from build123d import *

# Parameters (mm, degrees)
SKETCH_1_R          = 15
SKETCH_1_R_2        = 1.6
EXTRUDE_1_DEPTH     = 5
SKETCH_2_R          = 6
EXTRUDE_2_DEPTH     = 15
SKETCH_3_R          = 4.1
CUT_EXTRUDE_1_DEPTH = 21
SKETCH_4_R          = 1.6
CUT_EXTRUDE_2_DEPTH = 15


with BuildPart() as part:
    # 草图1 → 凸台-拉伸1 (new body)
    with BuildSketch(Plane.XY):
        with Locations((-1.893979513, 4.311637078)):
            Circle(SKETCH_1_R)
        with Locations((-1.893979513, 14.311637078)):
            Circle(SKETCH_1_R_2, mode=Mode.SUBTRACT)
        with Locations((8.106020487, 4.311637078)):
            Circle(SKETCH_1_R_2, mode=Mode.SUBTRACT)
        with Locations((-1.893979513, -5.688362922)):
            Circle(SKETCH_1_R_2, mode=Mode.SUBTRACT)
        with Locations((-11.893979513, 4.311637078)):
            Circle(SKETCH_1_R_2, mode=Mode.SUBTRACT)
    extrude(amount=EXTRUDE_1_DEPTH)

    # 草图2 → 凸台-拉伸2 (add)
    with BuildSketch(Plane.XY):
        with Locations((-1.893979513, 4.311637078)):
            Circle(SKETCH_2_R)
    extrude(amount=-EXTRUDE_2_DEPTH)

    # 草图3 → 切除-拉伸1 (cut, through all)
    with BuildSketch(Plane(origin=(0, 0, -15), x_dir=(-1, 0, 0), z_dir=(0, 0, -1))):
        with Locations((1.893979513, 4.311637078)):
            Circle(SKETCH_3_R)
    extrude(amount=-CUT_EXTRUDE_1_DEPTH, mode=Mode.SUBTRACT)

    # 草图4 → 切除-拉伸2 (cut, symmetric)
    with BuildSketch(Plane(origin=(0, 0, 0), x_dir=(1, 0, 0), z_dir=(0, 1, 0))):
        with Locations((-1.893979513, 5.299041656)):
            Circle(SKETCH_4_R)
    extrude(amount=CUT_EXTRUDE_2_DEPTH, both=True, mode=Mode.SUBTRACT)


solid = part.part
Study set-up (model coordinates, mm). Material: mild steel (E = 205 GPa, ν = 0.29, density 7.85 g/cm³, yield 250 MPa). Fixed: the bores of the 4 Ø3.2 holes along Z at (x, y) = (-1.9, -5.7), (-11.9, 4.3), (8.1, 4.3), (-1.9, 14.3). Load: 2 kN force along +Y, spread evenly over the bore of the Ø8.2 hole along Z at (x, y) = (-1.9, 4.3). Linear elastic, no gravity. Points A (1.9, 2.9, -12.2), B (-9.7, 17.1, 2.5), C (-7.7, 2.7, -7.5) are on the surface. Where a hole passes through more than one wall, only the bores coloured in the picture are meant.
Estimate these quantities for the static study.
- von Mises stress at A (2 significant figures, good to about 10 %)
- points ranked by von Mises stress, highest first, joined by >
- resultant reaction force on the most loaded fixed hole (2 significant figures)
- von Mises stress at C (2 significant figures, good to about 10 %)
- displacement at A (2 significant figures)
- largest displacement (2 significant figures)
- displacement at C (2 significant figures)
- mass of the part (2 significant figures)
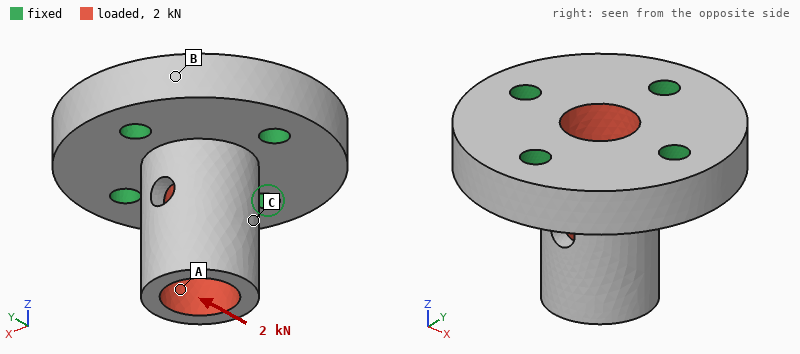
22 MPa
C > A > B
1.0 kN
43 MPa
12 µm
15 µm
7.5 µm
31 g
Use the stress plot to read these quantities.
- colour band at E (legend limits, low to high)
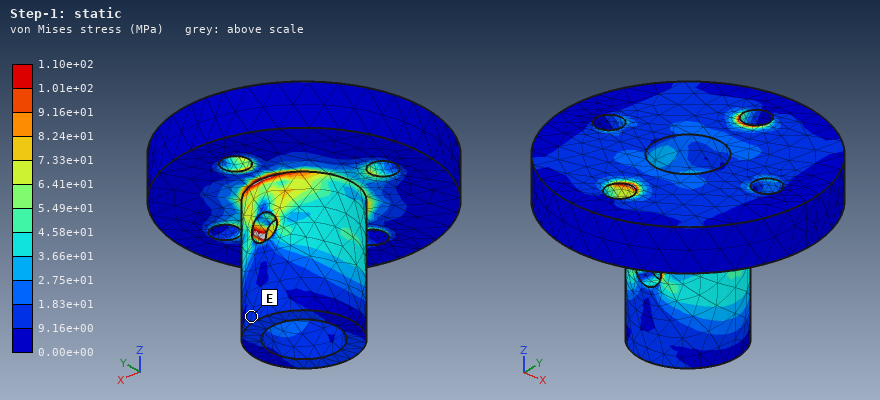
9.16e+00 to 1.83e+01 MPa
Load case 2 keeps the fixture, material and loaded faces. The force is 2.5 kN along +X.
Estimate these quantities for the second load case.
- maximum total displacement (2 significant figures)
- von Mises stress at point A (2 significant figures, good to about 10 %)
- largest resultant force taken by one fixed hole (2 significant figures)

19 µm
17 MPa
1.3 kN
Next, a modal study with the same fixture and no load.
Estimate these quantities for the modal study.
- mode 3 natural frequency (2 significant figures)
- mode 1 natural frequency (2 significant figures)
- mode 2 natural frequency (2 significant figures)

46 kHz
22 kHz
23 kHz
